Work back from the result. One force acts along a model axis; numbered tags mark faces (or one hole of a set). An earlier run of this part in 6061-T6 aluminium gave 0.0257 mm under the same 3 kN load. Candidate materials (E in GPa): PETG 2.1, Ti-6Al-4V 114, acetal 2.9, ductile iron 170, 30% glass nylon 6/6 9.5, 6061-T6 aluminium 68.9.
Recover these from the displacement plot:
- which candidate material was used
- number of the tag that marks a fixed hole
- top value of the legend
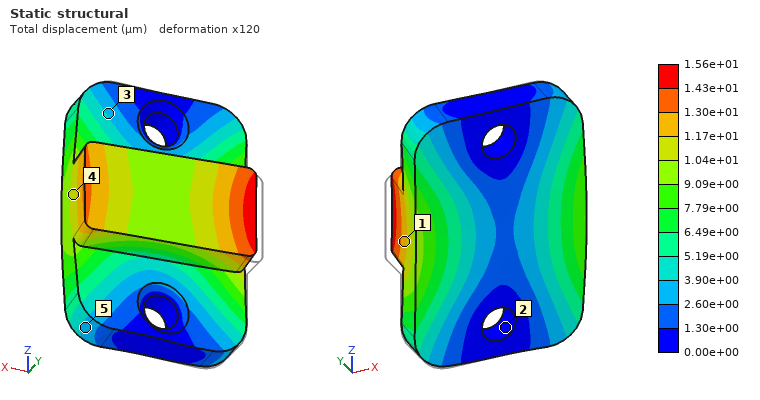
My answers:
Ti-6Al-4V
2
1.56e+01 µm
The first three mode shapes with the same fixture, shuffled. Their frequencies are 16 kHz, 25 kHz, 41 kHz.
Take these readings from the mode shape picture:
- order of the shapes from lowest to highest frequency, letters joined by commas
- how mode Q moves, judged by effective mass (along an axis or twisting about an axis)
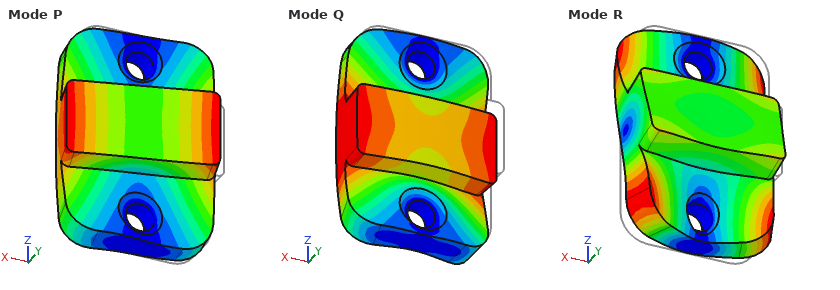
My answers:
P, Q, R
along Y
